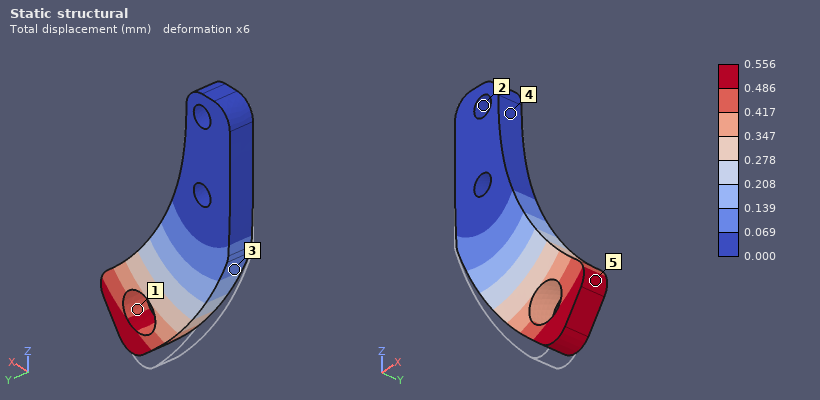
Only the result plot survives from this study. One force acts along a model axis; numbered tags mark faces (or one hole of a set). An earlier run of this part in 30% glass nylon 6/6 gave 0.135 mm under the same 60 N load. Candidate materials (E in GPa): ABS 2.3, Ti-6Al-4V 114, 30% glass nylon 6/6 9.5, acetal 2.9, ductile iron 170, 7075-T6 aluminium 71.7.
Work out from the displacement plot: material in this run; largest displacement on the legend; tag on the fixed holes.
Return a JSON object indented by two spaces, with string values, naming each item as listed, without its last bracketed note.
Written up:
{
  "material in this run": "ABS",
  "largest displacement on the legend": "0.556 mm",
  "tag on the fixed holes": "2"
}
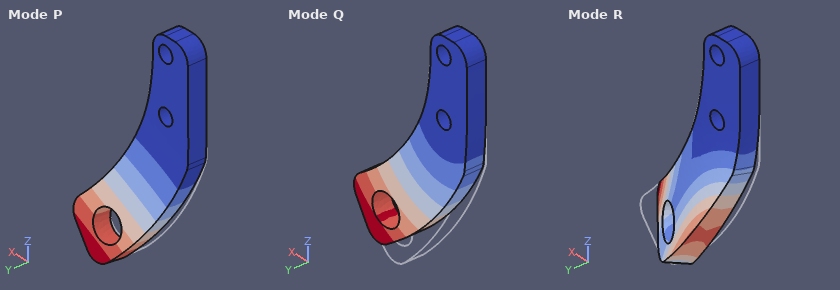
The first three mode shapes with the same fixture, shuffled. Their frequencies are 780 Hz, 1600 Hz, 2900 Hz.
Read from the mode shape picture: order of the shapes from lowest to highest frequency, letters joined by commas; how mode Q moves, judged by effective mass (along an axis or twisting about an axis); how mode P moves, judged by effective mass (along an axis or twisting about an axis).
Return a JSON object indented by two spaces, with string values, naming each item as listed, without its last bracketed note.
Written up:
{
  "order of the shapes from lowest to highest frequency, letters joined by commas": "P, Q, R",
  "how mode Q moves, judged by effective mass": "along X",
  "how mode P moves, judged by effective mass": "along Y"
}
